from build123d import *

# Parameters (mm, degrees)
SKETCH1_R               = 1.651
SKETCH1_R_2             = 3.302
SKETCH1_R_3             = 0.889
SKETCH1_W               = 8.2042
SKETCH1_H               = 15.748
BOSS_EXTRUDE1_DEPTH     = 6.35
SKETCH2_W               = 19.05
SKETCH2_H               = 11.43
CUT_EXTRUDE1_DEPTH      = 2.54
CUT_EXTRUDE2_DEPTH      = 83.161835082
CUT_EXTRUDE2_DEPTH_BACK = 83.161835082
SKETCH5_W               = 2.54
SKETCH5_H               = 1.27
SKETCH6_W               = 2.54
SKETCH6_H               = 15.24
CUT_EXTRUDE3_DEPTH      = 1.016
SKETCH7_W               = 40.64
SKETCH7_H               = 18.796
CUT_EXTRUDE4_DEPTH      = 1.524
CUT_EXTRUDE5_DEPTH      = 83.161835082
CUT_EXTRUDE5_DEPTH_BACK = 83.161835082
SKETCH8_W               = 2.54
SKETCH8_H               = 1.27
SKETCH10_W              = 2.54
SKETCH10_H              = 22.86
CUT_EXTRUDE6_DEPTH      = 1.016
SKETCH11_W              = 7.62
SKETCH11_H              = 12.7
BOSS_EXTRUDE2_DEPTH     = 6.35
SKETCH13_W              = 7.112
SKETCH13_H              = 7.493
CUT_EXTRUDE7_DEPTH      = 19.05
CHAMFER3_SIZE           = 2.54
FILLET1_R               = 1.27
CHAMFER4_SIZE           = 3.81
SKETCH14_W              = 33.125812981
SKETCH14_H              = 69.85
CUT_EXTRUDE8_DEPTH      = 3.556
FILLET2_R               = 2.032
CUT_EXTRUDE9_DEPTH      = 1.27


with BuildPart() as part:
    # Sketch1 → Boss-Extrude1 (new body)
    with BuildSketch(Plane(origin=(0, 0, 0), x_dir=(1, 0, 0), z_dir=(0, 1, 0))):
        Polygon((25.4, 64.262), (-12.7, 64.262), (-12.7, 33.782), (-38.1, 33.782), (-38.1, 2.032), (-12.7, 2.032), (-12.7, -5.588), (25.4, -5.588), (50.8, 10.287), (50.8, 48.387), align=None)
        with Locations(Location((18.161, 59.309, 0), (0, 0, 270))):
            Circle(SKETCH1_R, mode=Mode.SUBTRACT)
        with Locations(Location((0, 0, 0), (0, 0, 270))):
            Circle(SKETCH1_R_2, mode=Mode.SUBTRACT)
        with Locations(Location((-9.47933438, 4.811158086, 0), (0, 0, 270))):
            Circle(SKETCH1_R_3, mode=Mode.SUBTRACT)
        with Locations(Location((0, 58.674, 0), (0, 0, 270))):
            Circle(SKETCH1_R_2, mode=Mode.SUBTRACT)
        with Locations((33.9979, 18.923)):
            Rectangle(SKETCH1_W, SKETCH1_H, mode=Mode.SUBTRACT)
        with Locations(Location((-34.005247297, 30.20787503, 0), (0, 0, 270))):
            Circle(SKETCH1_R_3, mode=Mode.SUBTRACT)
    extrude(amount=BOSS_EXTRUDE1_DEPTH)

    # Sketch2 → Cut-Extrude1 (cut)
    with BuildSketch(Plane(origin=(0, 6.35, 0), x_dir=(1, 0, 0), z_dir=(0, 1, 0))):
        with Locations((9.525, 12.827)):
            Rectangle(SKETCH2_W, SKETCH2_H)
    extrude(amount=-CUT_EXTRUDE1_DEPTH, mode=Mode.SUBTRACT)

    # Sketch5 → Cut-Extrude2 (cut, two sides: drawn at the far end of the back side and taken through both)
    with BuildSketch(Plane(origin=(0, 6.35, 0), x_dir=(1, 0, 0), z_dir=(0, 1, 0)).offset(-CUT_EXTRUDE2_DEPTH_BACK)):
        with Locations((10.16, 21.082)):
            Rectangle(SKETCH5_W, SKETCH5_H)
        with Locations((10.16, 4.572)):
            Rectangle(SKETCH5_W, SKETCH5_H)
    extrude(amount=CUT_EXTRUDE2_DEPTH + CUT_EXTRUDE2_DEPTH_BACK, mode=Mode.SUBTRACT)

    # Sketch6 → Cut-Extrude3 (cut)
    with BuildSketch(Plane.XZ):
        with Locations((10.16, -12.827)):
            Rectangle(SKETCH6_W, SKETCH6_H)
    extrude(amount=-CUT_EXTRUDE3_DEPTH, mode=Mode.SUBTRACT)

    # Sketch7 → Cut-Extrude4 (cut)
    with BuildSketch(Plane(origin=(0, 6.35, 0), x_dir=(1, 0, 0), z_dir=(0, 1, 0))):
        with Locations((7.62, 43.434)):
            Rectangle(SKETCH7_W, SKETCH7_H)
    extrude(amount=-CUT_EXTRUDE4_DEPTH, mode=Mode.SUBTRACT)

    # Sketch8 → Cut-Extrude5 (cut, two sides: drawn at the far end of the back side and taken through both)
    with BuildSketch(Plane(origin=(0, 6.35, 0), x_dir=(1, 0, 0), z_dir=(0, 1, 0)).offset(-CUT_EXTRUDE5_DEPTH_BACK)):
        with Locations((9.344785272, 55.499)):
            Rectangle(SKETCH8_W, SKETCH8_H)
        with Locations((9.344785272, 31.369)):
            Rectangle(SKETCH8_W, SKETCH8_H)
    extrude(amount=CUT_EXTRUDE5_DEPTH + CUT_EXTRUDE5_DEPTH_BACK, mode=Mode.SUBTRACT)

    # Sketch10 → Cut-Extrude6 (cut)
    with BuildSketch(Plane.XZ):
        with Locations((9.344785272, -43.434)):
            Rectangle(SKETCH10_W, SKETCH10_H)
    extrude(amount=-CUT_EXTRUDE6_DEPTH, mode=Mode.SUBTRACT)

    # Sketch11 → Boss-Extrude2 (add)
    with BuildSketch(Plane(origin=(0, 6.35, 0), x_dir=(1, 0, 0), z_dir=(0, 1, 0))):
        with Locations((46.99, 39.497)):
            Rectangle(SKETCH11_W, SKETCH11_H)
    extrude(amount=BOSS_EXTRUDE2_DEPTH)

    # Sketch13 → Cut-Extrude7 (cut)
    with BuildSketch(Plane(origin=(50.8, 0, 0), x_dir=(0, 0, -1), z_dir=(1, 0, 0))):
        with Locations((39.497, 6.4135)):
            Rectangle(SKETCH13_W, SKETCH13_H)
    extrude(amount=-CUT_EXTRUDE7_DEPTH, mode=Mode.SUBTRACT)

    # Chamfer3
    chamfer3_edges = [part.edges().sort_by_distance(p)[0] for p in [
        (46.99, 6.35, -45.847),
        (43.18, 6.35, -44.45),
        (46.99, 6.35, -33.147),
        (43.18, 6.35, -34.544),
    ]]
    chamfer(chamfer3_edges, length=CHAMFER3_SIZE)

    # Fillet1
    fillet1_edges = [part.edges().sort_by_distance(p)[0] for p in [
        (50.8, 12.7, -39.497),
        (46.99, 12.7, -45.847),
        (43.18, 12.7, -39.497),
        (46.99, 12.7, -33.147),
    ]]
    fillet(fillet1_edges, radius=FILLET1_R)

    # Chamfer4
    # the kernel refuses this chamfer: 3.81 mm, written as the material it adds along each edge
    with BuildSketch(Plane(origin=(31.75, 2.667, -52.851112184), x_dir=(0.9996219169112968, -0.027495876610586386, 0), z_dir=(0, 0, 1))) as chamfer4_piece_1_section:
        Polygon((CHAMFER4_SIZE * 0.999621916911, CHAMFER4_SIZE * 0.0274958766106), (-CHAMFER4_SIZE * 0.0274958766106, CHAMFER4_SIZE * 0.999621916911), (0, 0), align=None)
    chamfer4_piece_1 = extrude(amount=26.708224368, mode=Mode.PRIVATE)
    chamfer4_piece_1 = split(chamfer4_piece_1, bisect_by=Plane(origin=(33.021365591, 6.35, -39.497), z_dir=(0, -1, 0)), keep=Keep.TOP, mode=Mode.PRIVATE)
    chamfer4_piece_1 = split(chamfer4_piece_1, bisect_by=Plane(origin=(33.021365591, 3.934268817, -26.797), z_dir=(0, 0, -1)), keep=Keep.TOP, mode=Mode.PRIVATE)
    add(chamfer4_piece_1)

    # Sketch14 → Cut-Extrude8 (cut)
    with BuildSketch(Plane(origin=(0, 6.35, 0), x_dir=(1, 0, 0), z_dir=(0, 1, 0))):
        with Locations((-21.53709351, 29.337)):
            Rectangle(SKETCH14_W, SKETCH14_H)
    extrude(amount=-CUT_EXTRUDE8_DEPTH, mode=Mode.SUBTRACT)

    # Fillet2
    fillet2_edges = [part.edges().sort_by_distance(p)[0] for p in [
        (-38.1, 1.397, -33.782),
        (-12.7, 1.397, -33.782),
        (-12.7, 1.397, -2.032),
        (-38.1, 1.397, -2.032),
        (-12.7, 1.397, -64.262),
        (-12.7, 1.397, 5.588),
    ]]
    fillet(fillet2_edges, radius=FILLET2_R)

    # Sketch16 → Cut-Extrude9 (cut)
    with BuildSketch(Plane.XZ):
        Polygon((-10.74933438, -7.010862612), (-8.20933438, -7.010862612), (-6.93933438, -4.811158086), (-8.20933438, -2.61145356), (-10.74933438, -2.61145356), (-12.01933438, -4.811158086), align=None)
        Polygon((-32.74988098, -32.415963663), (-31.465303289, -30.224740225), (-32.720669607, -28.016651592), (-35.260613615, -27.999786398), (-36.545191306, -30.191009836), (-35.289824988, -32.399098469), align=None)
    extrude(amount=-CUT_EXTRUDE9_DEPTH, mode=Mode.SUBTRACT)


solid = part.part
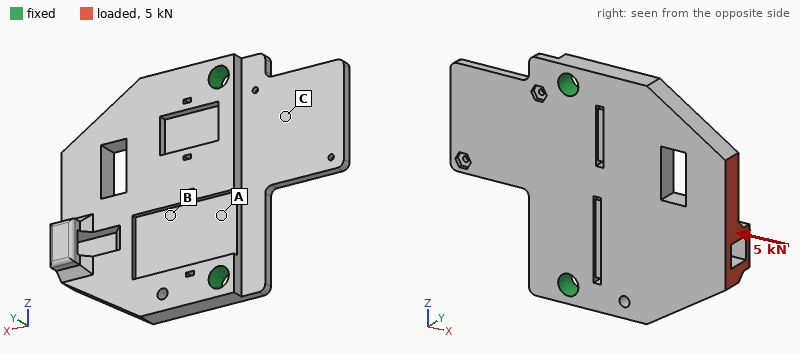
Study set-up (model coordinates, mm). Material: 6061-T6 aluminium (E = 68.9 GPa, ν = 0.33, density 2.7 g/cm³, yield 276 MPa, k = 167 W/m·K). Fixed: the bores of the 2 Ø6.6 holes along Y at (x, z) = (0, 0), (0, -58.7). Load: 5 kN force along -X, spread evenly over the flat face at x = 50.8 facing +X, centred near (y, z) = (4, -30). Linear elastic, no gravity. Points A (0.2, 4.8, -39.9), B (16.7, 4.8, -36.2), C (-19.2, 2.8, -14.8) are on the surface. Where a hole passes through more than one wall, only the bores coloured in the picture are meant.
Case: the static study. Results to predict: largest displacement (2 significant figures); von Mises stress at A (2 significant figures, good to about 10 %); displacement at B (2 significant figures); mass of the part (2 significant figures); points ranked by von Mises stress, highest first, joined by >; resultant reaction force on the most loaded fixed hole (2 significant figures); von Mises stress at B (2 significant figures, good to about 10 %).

0.14 mm
14 MPa
0.022 mm
62 g
B > A > C
2.7 kN
24 MPa
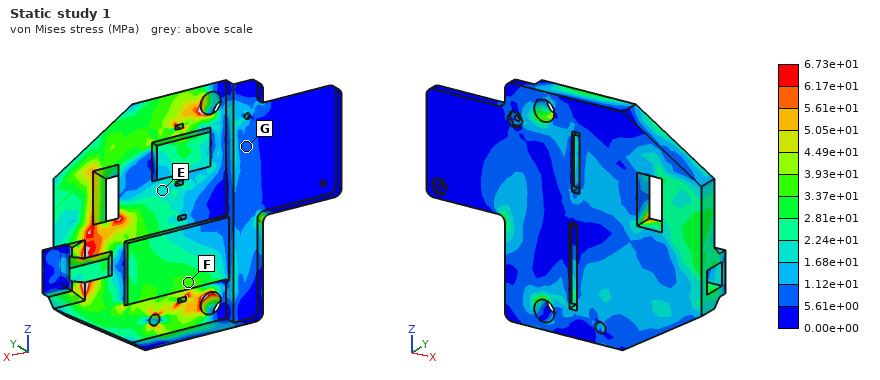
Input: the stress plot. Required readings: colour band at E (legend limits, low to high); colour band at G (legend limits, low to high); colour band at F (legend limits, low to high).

1.68e+01 to 2.24e+01 MPa
5.61e+00 to 1.12e+01 MPa
3.37e+01 to 3.93e+01 MPa
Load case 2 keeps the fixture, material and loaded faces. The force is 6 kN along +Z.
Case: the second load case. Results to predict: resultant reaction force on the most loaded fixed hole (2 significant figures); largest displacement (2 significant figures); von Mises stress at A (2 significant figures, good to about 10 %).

5.8 kN
0.11 mm
17 MPa
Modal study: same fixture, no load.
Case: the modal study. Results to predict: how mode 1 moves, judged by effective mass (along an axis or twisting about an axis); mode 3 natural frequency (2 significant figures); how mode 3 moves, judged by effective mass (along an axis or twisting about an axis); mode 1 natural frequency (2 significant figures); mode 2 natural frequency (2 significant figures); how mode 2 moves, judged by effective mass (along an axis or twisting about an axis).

along Y
4900 Hz
twisting about X
1700 Hz
2000 Hz
along Y
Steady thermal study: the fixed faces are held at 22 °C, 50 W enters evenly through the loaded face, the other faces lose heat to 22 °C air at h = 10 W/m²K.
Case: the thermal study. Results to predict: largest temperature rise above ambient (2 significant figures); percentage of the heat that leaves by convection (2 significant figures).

61 K
4.8 %
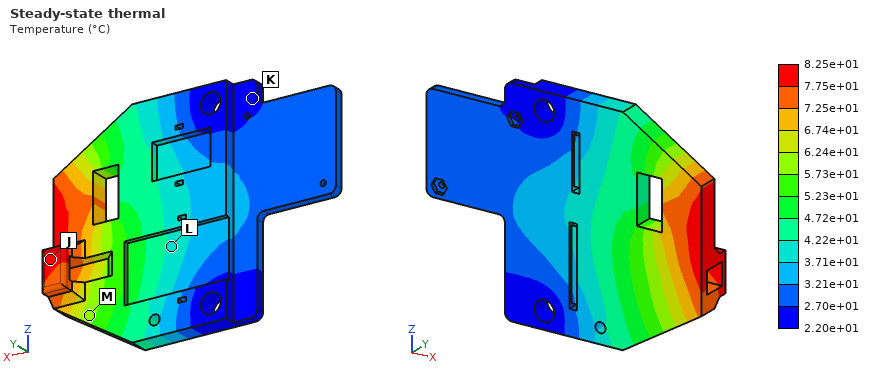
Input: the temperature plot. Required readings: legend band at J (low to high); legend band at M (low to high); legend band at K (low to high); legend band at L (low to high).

7.75e+01 to 8.25e+01 °C
5.73e+01 to 6.24e+01 °C
2.20e+01 to 2.70e+01 °C
3.71e+01 to 4.22e+01 °C
